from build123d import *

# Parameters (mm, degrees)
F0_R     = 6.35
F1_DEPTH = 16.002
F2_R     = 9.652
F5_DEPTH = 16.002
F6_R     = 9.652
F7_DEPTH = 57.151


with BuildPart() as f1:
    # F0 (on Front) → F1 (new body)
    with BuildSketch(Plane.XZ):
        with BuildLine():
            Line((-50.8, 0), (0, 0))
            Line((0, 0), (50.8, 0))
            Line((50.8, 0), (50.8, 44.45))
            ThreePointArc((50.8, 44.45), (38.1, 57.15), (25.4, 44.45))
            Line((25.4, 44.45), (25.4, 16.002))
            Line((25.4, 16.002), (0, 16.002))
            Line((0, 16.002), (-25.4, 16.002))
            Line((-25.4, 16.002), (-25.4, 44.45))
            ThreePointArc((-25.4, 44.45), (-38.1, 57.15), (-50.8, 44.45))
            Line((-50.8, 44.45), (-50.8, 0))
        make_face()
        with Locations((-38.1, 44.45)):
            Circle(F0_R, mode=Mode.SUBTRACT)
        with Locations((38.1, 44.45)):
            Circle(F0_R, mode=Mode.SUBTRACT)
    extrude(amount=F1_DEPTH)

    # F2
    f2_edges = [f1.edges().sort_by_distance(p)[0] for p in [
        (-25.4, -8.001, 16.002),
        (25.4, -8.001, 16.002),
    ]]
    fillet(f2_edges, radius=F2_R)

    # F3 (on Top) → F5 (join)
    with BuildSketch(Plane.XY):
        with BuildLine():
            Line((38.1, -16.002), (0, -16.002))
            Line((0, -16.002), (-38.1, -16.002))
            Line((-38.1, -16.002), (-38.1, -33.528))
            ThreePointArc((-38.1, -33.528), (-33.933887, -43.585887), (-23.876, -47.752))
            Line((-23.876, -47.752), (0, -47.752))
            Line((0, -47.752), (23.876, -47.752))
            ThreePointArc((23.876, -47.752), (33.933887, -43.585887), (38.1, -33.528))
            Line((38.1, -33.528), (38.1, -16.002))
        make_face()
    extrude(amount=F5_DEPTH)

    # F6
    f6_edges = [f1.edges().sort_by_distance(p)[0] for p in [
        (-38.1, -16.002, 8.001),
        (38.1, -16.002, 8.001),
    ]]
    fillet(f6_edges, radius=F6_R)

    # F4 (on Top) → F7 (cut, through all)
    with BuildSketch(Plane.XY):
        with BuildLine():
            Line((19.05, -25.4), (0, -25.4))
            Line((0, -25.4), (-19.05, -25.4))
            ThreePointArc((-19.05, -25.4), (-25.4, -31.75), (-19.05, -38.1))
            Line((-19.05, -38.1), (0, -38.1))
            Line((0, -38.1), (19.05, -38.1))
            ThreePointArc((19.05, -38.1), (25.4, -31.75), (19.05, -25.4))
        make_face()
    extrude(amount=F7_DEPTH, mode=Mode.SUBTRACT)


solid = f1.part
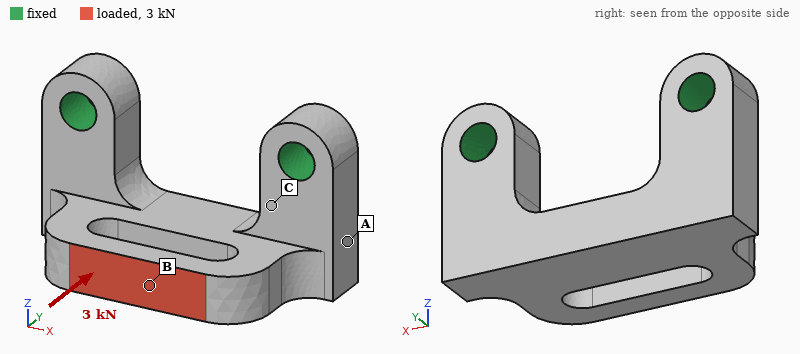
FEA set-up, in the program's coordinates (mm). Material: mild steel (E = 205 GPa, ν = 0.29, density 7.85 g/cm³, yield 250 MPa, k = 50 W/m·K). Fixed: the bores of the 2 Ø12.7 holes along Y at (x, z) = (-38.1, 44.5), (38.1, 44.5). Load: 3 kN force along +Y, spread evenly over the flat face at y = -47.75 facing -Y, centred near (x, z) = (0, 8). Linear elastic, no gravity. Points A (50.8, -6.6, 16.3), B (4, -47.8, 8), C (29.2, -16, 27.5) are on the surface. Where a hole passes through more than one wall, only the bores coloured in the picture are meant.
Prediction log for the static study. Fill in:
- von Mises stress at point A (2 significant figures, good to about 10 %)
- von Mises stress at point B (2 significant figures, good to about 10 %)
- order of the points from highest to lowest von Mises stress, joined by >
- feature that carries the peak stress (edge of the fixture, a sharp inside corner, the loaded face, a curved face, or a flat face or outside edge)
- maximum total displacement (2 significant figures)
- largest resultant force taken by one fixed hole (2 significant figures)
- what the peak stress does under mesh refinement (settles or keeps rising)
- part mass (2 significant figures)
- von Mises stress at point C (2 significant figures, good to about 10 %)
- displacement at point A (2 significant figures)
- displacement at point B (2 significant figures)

10 MPa
39 MPa
B > C > A
edge of the fixture
33 µm
1.5 kN
keeps rising
640 g
28 MPa
7.1 µm
29 µm
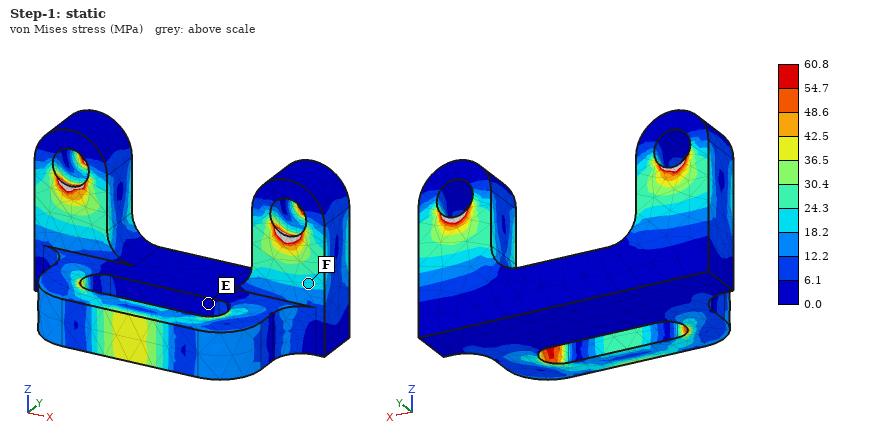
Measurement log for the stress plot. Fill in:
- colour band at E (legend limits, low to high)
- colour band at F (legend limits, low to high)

0.0 to 6.1 MPa
18.2 to 24.3 MPa
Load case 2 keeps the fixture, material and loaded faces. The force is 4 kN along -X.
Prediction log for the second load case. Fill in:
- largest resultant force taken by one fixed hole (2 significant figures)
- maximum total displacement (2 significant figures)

2.8 kN
24 µm
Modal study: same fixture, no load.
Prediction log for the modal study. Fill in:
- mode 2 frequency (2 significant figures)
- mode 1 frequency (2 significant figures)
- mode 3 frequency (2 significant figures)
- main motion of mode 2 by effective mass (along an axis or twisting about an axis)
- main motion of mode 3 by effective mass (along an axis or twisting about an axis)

5200 Hz
2900 Hz
6600 Hz
along X
along Y
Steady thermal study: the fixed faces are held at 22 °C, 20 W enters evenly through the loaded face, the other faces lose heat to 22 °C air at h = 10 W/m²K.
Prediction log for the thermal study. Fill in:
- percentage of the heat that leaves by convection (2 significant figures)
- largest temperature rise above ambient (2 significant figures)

14 %
54 K
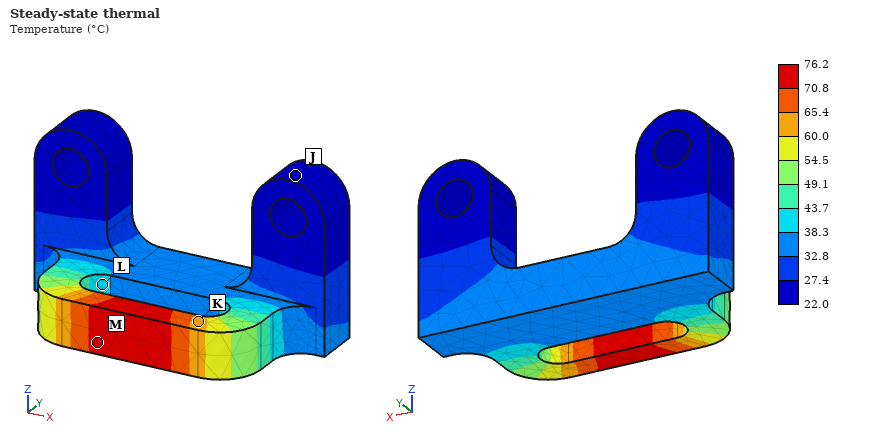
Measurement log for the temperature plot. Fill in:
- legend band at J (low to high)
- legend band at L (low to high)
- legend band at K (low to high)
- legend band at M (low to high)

22.0 to 27.4 °C
38.3 to 43.7 °C
60.0 to 65.4 °C
70.8 to 76.2 °C
